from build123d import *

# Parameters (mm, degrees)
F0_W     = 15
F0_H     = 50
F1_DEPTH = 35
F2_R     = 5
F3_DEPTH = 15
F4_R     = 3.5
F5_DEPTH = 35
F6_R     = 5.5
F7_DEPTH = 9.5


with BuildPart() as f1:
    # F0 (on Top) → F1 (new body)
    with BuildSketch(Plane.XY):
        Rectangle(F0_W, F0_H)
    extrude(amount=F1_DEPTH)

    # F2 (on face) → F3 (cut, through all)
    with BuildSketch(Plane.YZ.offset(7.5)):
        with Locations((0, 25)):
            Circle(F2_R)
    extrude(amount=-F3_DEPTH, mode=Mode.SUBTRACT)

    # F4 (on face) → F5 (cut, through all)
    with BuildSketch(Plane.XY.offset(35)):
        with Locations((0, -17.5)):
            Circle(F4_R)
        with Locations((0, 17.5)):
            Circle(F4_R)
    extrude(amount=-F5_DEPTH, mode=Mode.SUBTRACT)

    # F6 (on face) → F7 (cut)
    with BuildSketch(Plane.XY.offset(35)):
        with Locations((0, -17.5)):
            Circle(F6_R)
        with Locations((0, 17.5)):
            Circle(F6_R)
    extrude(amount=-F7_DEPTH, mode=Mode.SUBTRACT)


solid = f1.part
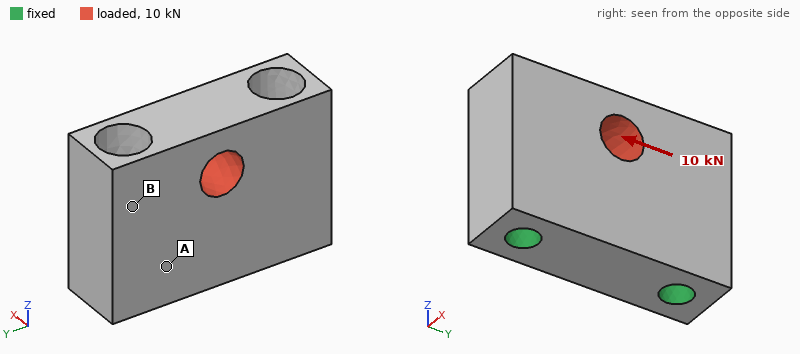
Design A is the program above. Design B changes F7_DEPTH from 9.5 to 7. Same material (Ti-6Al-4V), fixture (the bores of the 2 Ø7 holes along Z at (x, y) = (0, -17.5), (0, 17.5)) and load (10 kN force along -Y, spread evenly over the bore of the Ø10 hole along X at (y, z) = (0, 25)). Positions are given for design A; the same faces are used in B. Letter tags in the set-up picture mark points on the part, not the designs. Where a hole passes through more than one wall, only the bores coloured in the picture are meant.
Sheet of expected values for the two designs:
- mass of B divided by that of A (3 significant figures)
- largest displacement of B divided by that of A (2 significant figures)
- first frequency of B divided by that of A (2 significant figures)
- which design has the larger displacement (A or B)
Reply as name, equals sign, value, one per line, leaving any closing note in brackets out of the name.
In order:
mass of B divided by that of A = 1.01
largest displacement of B divided by that of A = 0.76
first frequency of B divided by that of A = 1.2
which design has the larger displacement = A
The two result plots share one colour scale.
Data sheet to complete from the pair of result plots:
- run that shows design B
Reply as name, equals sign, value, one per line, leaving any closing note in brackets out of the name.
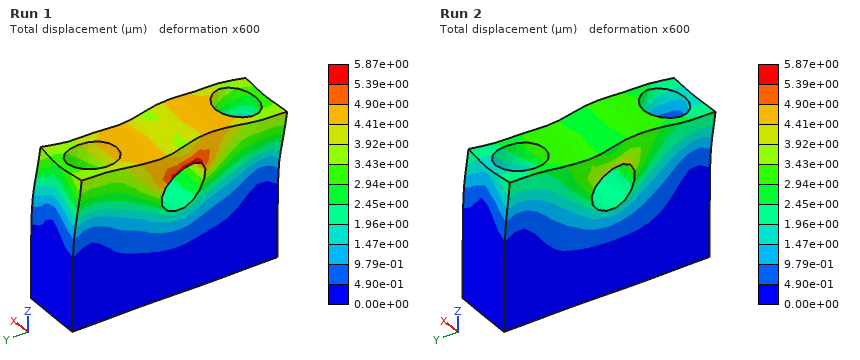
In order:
run that shows design B = Run 2
